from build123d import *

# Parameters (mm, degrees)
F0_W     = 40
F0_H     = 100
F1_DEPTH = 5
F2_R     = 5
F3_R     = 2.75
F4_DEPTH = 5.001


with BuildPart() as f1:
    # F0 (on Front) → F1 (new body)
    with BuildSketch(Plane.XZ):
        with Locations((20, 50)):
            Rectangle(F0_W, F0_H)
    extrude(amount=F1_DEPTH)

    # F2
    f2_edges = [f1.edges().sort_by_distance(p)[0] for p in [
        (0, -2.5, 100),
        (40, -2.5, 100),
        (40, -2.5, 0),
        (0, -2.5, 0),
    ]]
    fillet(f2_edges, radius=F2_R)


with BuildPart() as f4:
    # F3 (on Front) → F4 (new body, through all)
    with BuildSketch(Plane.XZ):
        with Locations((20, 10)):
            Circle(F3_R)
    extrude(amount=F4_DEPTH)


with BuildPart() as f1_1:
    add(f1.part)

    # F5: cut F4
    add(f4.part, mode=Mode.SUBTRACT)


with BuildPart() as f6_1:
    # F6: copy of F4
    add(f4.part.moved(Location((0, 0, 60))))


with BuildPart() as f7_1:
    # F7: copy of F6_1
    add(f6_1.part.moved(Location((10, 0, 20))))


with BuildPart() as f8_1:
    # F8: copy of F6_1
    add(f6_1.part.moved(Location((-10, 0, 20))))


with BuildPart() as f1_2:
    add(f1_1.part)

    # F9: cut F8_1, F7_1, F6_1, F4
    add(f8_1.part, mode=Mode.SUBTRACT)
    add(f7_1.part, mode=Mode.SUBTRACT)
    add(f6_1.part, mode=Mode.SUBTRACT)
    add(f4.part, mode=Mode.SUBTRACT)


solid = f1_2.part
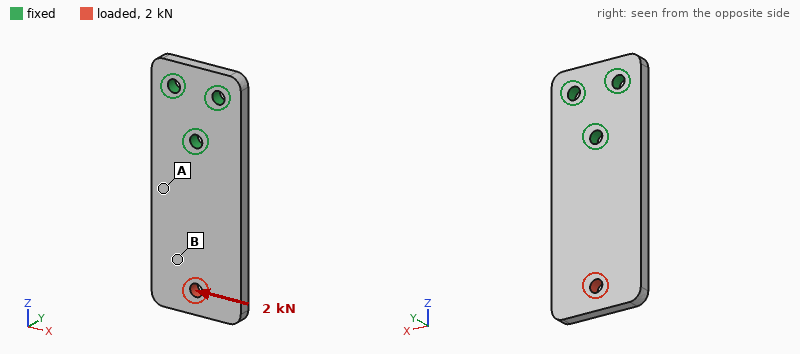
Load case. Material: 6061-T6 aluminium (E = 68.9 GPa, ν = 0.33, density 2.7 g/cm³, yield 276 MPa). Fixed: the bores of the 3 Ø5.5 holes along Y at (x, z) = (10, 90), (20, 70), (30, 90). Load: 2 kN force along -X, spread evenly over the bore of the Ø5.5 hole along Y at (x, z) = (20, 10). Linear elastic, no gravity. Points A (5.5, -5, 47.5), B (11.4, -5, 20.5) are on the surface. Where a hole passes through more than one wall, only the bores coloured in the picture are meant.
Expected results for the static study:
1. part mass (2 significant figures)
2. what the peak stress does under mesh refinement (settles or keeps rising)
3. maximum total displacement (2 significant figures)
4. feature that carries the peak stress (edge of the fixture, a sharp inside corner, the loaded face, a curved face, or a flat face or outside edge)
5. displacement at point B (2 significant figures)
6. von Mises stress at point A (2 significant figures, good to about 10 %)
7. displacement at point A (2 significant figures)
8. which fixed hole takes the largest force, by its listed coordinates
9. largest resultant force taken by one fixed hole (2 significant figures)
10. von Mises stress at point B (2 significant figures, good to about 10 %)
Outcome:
52 g
keeps rising
0.21 mm
edge of the fixture
0.14 mm
43 MPa
0.061 mm
(20, 70)
4.2 kN
22 MPa
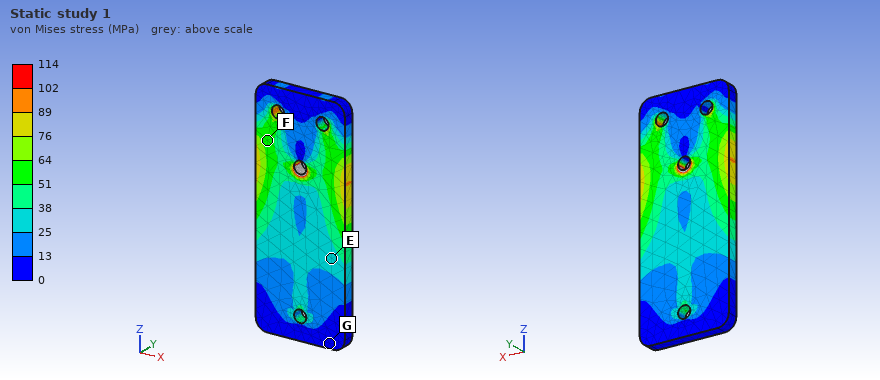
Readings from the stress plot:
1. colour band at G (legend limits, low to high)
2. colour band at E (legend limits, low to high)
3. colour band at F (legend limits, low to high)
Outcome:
0 to 13 MPa
25 to 38 MPa
51 to 64 MPa
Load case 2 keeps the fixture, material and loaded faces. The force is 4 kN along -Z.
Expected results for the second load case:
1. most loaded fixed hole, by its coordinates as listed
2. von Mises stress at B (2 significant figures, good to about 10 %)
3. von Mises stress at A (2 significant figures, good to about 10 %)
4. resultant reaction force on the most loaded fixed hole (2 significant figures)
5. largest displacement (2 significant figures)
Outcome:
(20, 70)
26 MPa
19 MPa
2.5 kN
28 µm
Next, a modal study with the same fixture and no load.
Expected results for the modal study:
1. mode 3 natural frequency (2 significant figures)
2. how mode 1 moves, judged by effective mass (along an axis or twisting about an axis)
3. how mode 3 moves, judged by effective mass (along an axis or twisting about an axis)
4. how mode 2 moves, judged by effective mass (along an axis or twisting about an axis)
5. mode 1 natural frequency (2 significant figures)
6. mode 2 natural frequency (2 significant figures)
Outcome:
4200 Hz
along Y
along X
twisting about Z
850 Hz
2700 Hz
